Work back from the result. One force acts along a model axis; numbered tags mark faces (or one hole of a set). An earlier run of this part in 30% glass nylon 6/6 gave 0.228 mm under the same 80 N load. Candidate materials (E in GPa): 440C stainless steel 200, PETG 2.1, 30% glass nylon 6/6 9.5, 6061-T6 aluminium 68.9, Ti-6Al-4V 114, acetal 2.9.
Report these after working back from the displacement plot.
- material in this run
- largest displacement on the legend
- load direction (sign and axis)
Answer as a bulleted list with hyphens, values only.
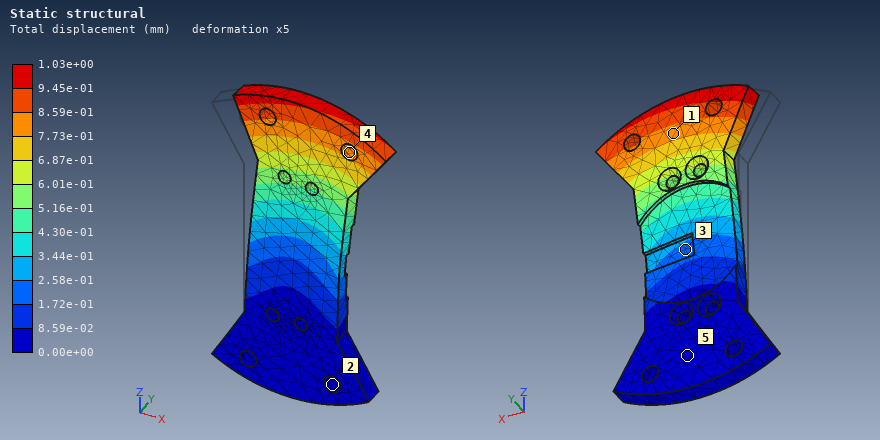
- PETG
- 1.03e+00 mm
- +X
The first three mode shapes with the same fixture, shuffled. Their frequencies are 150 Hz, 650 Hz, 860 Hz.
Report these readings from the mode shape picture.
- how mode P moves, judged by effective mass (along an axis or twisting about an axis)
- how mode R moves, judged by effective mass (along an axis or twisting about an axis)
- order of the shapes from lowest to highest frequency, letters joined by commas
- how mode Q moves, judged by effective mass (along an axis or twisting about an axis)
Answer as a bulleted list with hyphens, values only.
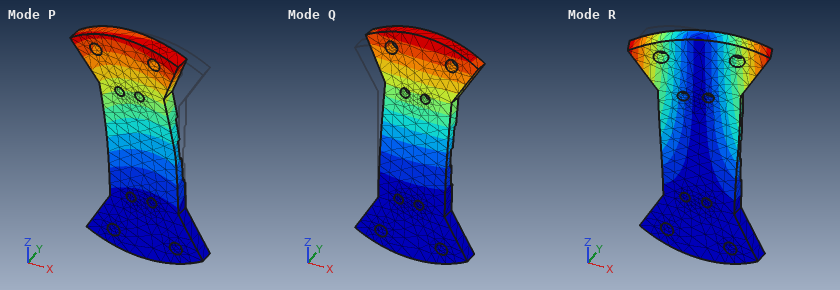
- along X
- twisting about Z
- Q, R, P
- along Y
